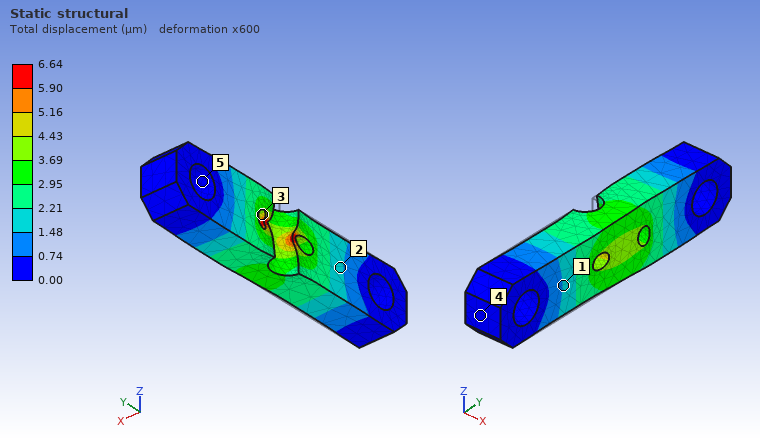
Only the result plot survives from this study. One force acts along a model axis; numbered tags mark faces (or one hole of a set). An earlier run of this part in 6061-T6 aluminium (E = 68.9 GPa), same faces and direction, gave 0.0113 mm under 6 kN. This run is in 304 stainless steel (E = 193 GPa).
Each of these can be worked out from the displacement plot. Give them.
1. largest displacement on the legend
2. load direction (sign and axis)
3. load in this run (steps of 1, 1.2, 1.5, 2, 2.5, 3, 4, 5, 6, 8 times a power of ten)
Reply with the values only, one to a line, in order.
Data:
6.64 µm
+Y
10 kN
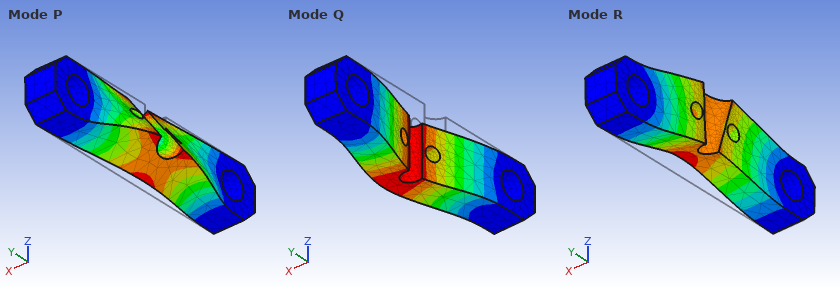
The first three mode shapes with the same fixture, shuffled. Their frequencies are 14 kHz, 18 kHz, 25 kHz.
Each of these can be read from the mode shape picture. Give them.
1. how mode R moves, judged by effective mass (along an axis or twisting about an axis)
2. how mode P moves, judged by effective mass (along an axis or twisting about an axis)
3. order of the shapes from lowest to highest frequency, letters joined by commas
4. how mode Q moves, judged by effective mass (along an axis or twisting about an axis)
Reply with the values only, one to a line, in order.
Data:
along Z
twisting about Y
Q, R, P
along X
